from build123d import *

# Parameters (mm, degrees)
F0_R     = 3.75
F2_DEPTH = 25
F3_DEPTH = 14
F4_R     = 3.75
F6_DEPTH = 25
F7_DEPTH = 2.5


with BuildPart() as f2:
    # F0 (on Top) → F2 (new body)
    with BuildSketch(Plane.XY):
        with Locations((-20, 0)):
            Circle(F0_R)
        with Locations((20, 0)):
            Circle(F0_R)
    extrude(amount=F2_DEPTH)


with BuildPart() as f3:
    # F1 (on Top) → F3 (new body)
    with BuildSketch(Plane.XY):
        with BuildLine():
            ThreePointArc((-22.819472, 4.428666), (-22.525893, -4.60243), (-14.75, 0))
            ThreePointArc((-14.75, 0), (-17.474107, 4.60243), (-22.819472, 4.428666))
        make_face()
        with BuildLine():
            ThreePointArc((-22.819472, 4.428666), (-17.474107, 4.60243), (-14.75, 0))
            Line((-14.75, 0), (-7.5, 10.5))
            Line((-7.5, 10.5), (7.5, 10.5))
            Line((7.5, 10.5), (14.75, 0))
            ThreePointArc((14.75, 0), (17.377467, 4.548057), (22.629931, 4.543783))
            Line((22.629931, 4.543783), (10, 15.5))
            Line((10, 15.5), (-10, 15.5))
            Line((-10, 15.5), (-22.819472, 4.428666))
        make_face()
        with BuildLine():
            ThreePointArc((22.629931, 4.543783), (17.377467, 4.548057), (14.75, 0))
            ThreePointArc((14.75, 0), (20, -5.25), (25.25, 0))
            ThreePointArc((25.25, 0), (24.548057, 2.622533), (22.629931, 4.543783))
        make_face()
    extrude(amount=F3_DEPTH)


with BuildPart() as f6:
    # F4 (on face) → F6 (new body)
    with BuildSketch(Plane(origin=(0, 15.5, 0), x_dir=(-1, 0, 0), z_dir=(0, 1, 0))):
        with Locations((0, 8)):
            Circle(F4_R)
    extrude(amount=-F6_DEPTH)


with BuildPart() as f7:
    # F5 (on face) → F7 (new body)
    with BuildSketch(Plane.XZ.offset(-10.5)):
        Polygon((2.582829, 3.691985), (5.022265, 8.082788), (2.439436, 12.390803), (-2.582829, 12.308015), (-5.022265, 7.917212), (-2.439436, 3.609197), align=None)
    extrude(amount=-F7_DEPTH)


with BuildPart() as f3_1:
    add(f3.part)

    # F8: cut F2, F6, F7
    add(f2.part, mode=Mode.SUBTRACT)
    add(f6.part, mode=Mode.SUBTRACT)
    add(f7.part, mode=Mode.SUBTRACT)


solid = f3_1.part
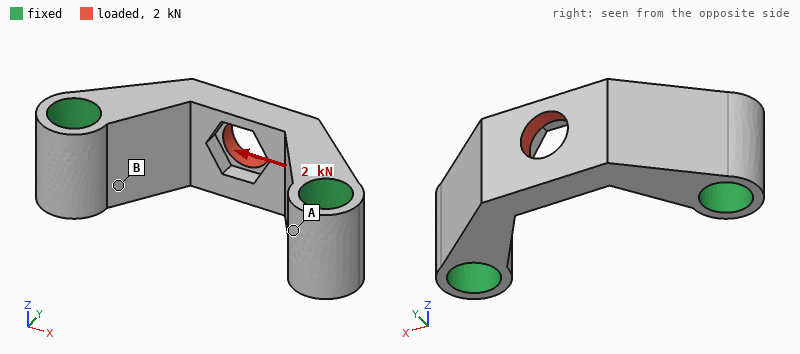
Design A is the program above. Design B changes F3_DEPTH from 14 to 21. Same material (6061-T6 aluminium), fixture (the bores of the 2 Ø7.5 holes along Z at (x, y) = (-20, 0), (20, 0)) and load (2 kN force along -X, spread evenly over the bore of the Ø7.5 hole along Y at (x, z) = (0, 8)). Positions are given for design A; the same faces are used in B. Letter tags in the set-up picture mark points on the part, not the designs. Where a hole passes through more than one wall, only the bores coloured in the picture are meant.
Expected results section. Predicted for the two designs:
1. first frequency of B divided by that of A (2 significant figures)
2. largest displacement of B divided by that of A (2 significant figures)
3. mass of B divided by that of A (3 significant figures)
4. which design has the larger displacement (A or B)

1.1
0.75
1.53
A
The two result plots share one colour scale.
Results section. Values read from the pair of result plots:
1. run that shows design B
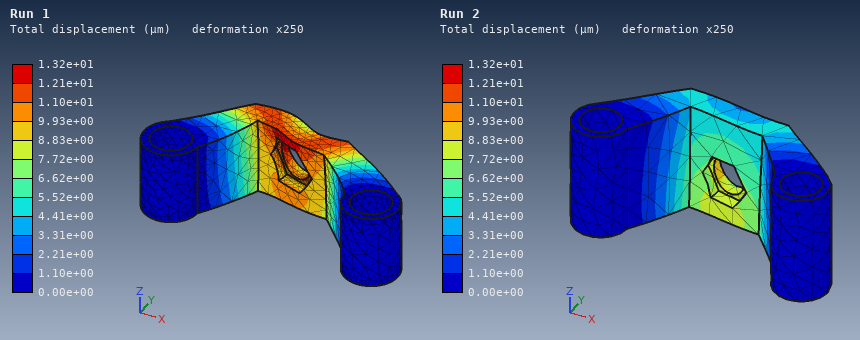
Run 2
